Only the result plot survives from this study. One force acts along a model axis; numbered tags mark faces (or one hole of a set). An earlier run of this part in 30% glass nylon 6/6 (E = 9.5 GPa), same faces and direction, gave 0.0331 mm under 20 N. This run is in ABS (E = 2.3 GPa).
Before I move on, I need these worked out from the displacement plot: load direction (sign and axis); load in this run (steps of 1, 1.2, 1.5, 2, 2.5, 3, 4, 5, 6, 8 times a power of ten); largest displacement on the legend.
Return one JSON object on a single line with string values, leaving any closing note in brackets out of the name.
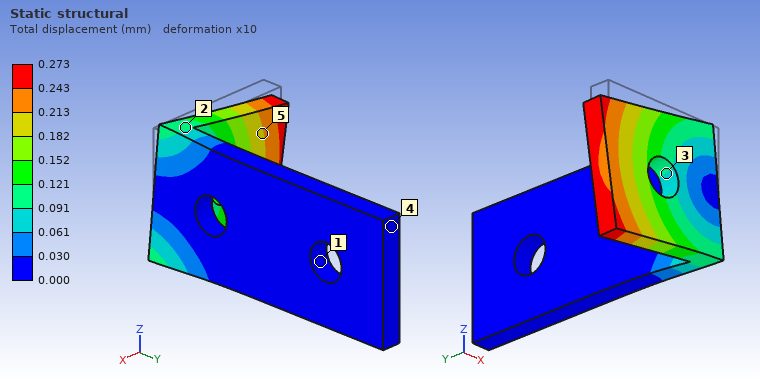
{"load direction": "-Z", "load in this run": "40 N", "largest displacement on the legend": "0.273 mm"}
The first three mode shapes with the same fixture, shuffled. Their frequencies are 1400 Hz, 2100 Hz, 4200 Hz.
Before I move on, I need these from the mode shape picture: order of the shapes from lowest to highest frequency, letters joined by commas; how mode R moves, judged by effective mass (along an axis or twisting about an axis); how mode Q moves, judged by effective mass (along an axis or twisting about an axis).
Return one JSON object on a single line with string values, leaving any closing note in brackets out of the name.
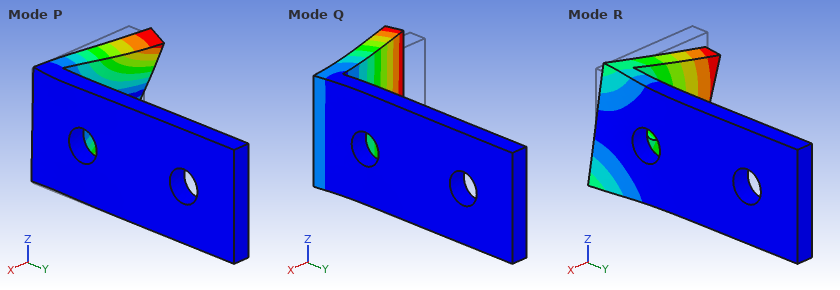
{"order of the shapes from lowest to highest frequency, letters joined by commas": "Q, R, P", "how mode R moves, judged by effective mass": "along Z", "how mode Q moves, judged by effective mass": "along Y"}
